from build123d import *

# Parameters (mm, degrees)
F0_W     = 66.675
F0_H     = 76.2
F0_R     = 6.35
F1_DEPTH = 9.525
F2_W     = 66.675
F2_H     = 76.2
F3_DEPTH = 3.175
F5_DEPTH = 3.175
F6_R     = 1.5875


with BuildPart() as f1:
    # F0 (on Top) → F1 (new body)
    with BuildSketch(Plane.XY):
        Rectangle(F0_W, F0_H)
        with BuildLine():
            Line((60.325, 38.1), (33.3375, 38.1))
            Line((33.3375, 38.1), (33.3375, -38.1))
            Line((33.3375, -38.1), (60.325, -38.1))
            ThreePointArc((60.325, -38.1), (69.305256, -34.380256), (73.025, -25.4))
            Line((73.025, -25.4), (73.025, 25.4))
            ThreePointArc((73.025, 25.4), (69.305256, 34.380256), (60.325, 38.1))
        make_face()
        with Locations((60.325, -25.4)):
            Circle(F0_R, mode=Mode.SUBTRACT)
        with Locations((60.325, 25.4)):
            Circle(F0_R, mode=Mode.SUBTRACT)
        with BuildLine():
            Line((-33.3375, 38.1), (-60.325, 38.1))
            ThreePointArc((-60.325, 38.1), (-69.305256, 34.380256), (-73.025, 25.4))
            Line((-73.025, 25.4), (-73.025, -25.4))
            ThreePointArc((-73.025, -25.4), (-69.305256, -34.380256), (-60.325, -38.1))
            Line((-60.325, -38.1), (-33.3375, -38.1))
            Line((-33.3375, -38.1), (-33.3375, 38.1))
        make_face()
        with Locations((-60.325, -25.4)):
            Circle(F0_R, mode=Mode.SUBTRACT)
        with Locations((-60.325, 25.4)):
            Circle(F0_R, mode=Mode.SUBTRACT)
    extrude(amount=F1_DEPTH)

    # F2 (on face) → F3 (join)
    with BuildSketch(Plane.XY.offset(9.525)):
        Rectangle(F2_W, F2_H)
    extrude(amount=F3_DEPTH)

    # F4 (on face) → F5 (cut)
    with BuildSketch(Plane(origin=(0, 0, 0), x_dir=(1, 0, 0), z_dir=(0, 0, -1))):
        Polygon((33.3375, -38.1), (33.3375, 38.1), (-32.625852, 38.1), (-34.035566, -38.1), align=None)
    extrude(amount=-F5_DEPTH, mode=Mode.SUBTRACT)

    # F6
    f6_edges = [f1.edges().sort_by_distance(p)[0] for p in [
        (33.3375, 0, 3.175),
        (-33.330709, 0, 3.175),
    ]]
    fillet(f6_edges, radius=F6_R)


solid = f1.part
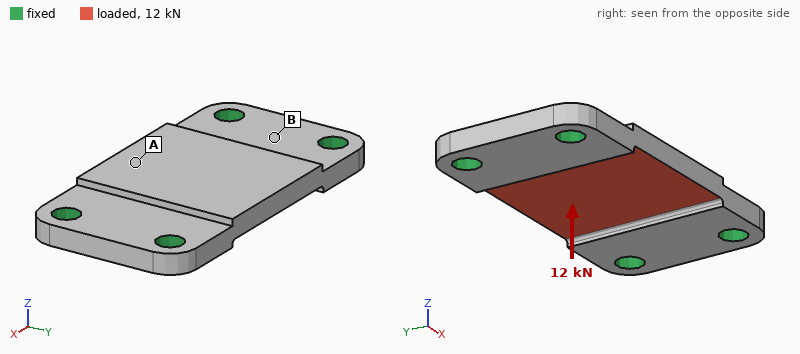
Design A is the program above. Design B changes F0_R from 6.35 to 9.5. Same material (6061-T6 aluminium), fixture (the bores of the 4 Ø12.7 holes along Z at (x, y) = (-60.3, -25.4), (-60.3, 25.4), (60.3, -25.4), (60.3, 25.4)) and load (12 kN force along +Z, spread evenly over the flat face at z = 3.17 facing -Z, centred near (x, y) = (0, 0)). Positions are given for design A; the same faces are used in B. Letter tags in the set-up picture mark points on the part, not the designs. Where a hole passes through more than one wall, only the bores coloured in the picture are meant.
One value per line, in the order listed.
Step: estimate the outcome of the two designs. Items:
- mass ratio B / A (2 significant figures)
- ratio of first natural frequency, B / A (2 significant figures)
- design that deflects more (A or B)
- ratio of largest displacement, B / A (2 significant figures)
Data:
0.94
1.1
A
0.81
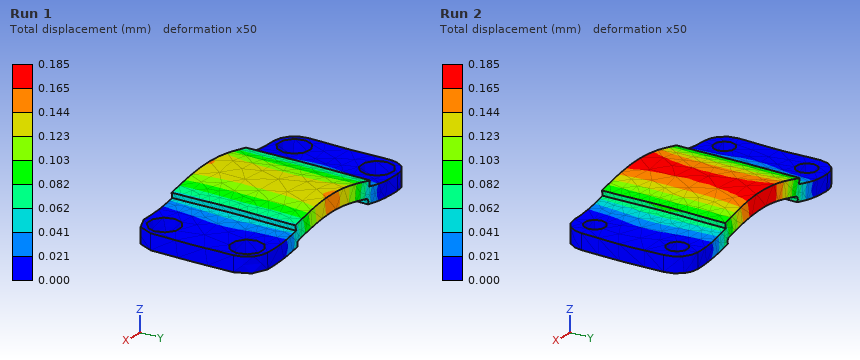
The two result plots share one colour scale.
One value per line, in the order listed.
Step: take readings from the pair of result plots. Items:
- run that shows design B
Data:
Run 1
